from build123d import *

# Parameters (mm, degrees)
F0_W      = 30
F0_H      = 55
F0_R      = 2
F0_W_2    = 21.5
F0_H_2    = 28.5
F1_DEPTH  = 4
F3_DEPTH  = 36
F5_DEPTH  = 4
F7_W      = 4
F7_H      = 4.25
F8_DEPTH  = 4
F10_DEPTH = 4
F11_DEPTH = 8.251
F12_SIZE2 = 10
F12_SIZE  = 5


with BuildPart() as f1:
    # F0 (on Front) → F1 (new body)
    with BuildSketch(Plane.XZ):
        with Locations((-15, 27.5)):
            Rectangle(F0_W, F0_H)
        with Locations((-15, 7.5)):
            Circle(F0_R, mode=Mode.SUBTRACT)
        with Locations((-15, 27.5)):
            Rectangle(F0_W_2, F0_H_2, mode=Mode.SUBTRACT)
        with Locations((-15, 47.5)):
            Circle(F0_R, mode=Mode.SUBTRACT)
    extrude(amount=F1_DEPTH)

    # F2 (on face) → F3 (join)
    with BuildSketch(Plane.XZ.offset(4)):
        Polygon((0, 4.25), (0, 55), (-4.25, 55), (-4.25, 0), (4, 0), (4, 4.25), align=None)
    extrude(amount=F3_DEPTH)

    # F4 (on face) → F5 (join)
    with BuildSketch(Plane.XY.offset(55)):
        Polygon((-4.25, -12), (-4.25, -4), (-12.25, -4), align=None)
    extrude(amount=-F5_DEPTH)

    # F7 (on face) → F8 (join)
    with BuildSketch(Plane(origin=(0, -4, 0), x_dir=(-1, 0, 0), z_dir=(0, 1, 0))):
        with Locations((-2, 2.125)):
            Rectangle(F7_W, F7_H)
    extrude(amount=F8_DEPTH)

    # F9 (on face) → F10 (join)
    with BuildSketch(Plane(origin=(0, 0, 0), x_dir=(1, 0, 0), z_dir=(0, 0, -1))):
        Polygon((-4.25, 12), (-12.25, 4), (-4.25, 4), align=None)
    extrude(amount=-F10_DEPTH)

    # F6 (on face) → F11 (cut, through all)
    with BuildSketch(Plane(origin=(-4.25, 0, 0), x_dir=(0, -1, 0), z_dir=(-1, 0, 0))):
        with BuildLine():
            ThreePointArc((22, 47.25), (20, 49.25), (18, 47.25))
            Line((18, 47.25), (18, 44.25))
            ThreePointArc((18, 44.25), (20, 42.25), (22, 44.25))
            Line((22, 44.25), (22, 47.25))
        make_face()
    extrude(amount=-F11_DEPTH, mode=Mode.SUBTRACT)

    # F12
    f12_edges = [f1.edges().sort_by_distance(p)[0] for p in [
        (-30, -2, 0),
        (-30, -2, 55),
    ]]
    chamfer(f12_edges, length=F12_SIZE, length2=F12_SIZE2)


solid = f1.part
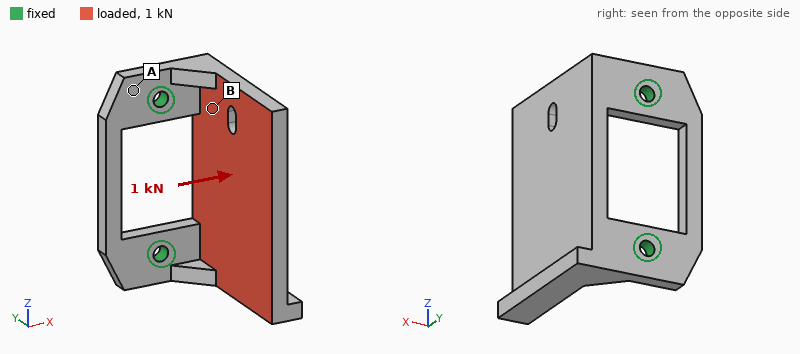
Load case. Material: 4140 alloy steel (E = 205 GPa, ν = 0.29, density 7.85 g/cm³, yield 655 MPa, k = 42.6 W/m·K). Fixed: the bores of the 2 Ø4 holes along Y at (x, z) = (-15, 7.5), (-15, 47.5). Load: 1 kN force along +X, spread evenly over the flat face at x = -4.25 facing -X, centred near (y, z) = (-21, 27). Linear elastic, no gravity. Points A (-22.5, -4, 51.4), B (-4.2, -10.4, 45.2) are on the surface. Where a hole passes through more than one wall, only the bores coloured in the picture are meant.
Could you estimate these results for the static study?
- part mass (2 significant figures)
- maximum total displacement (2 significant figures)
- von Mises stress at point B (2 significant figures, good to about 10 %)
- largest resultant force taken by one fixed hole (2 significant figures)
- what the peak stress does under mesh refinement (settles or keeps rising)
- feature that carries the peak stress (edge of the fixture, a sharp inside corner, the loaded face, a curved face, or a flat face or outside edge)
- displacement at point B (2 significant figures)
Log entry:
100 g
0.26 mm
61 MPa
560 N
keeps rising
edge of the fixture
0.050 mm
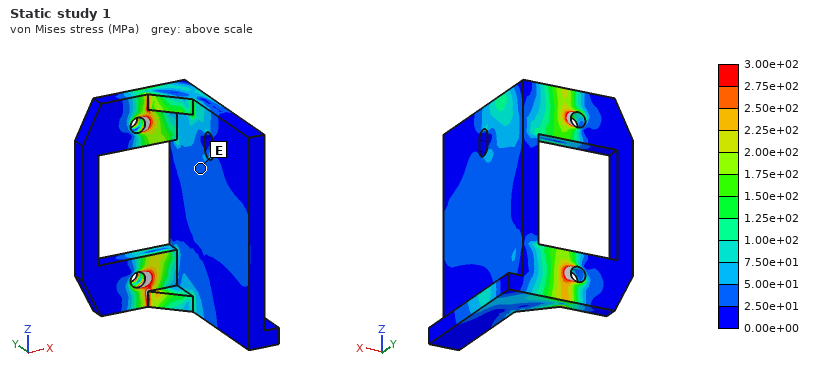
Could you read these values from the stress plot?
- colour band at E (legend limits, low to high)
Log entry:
2.50e+01 to 5.00e+01 MPa
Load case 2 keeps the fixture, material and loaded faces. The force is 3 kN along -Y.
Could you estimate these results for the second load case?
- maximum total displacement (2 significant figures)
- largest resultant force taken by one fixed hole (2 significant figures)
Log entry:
0.16 mm
1.5 kN
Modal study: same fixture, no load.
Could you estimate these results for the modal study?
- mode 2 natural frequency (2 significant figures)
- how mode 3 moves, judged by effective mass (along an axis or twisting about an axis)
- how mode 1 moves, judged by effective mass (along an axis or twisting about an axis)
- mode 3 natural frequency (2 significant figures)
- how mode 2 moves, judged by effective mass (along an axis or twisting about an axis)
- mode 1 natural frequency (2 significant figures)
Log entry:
3200 Hz
along Z
along X
5400 Hz
along Z
1400 Hz
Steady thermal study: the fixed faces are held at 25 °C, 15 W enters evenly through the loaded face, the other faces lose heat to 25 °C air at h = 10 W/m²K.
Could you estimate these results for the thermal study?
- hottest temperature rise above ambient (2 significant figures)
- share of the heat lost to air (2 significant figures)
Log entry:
60 K
12 %
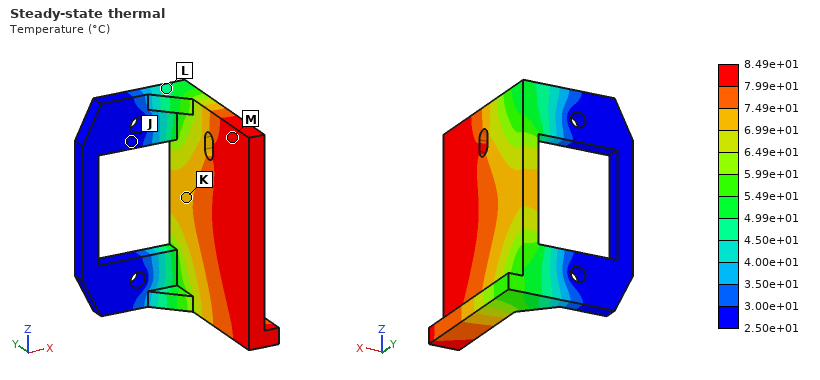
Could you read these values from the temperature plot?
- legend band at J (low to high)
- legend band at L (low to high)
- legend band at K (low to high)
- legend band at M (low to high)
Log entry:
2.50e+01 to 3.00e+01 °C
4.50e+01 to 4.99e+01 °C
6.99e+01 to 7.49e+01 °C
7.99e+01 to 8.49e+01 °C
